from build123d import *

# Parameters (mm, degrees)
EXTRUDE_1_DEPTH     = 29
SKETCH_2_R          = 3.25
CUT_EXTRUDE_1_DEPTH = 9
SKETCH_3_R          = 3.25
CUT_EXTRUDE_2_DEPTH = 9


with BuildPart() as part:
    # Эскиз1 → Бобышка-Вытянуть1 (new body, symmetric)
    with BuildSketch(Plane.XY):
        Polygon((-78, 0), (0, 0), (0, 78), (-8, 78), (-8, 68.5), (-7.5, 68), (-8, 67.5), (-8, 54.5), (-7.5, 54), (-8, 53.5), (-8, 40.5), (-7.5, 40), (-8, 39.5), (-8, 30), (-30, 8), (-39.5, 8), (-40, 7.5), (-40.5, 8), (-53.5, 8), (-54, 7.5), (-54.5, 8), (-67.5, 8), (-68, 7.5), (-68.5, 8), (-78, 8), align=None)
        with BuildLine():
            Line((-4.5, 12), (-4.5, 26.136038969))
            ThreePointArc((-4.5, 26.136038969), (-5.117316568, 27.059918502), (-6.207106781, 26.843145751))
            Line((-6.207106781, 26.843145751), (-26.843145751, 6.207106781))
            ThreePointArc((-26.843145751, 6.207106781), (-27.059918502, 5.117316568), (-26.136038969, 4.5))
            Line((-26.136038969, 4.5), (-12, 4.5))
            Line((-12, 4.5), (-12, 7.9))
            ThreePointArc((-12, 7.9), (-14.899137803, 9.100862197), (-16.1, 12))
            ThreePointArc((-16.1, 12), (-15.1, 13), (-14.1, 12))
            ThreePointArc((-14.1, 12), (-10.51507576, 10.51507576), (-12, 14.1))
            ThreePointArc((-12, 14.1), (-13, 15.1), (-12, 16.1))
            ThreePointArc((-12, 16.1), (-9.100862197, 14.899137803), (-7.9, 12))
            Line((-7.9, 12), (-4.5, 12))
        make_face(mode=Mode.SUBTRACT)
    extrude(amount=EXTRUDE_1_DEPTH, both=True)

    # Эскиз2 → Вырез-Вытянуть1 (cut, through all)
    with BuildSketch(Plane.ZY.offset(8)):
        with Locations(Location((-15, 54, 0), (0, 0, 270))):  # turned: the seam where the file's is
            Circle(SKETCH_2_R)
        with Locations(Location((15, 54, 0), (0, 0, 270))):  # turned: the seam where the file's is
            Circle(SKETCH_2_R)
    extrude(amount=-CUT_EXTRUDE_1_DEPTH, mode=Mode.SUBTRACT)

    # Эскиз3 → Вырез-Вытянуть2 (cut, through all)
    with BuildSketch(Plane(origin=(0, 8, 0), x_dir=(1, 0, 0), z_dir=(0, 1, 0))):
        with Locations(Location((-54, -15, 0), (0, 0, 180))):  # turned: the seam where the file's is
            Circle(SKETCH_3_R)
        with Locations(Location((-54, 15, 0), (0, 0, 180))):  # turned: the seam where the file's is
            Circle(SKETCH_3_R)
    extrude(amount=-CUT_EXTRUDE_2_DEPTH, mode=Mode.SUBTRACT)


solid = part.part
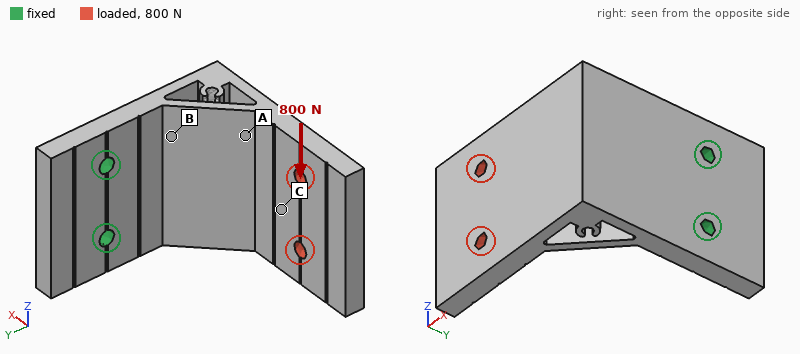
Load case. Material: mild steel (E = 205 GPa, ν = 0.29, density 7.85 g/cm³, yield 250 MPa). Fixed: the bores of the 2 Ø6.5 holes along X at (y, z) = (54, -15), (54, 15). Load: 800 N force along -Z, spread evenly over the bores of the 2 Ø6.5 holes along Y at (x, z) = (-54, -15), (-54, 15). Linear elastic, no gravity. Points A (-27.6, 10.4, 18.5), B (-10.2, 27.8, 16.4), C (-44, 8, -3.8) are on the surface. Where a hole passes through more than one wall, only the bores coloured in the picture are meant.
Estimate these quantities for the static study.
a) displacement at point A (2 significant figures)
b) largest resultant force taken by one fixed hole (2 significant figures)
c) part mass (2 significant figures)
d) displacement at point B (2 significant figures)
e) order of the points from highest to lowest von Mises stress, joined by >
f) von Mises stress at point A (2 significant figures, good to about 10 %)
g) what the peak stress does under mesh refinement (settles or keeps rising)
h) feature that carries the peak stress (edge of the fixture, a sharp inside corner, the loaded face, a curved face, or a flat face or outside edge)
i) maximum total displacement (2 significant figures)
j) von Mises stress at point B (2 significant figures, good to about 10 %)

23 µm
1.6 kN
540 g
11 µm
B > A > C
13 MPa
keeps rising
edge of the fixture
61 µm
28 MPa
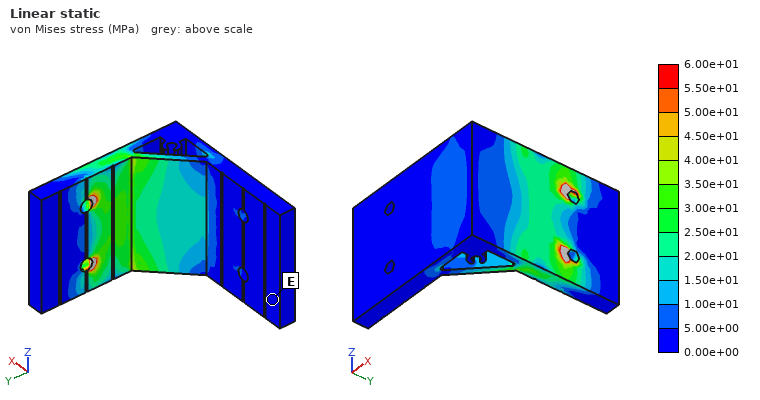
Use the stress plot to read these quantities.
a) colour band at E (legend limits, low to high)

0.00e+00 to 5.00e+00 MPa
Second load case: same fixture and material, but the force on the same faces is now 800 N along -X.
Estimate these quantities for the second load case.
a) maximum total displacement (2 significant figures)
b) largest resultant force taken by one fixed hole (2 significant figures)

0.18 mm
400 N
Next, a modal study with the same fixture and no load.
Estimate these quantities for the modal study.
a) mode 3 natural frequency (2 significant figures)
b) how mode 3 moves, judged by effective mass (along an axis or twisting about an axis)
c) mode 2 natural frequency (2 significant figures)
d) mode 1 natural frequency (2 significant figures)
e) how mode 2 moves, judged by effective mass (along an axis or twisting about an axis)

2300 Hz
along X
1500 Hz
600 Hz
along Z
